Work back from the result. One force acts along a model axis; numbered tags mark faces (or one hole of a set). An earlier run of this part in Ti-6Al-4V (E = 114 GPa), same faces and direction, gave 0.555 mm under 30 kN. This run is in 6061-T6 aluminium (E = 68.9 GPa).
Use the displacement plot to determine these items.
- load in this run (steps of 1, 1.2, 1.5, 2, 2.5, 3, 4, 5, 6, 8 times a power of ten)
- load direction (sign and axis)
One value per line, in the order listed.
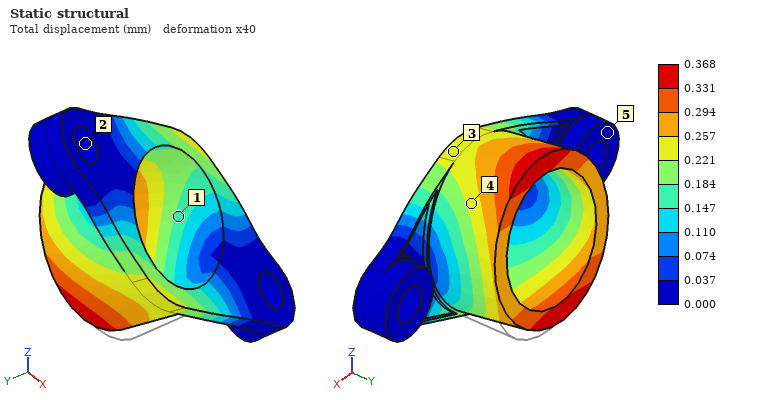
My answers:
12 kN
+Z
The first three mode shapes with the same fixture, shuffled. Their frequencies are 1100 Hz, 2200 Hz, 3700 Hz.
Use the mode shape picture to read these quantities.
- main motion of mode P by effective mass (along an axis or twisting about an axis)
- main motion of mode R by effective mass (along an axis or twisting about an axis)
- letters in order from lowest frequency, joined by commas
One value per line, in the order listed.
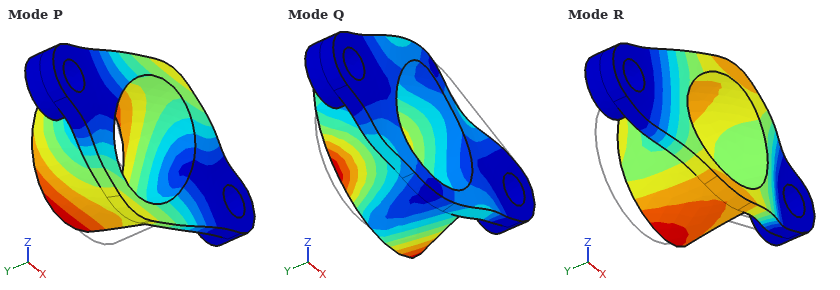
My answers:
along Z
along Y
P, R, Q
